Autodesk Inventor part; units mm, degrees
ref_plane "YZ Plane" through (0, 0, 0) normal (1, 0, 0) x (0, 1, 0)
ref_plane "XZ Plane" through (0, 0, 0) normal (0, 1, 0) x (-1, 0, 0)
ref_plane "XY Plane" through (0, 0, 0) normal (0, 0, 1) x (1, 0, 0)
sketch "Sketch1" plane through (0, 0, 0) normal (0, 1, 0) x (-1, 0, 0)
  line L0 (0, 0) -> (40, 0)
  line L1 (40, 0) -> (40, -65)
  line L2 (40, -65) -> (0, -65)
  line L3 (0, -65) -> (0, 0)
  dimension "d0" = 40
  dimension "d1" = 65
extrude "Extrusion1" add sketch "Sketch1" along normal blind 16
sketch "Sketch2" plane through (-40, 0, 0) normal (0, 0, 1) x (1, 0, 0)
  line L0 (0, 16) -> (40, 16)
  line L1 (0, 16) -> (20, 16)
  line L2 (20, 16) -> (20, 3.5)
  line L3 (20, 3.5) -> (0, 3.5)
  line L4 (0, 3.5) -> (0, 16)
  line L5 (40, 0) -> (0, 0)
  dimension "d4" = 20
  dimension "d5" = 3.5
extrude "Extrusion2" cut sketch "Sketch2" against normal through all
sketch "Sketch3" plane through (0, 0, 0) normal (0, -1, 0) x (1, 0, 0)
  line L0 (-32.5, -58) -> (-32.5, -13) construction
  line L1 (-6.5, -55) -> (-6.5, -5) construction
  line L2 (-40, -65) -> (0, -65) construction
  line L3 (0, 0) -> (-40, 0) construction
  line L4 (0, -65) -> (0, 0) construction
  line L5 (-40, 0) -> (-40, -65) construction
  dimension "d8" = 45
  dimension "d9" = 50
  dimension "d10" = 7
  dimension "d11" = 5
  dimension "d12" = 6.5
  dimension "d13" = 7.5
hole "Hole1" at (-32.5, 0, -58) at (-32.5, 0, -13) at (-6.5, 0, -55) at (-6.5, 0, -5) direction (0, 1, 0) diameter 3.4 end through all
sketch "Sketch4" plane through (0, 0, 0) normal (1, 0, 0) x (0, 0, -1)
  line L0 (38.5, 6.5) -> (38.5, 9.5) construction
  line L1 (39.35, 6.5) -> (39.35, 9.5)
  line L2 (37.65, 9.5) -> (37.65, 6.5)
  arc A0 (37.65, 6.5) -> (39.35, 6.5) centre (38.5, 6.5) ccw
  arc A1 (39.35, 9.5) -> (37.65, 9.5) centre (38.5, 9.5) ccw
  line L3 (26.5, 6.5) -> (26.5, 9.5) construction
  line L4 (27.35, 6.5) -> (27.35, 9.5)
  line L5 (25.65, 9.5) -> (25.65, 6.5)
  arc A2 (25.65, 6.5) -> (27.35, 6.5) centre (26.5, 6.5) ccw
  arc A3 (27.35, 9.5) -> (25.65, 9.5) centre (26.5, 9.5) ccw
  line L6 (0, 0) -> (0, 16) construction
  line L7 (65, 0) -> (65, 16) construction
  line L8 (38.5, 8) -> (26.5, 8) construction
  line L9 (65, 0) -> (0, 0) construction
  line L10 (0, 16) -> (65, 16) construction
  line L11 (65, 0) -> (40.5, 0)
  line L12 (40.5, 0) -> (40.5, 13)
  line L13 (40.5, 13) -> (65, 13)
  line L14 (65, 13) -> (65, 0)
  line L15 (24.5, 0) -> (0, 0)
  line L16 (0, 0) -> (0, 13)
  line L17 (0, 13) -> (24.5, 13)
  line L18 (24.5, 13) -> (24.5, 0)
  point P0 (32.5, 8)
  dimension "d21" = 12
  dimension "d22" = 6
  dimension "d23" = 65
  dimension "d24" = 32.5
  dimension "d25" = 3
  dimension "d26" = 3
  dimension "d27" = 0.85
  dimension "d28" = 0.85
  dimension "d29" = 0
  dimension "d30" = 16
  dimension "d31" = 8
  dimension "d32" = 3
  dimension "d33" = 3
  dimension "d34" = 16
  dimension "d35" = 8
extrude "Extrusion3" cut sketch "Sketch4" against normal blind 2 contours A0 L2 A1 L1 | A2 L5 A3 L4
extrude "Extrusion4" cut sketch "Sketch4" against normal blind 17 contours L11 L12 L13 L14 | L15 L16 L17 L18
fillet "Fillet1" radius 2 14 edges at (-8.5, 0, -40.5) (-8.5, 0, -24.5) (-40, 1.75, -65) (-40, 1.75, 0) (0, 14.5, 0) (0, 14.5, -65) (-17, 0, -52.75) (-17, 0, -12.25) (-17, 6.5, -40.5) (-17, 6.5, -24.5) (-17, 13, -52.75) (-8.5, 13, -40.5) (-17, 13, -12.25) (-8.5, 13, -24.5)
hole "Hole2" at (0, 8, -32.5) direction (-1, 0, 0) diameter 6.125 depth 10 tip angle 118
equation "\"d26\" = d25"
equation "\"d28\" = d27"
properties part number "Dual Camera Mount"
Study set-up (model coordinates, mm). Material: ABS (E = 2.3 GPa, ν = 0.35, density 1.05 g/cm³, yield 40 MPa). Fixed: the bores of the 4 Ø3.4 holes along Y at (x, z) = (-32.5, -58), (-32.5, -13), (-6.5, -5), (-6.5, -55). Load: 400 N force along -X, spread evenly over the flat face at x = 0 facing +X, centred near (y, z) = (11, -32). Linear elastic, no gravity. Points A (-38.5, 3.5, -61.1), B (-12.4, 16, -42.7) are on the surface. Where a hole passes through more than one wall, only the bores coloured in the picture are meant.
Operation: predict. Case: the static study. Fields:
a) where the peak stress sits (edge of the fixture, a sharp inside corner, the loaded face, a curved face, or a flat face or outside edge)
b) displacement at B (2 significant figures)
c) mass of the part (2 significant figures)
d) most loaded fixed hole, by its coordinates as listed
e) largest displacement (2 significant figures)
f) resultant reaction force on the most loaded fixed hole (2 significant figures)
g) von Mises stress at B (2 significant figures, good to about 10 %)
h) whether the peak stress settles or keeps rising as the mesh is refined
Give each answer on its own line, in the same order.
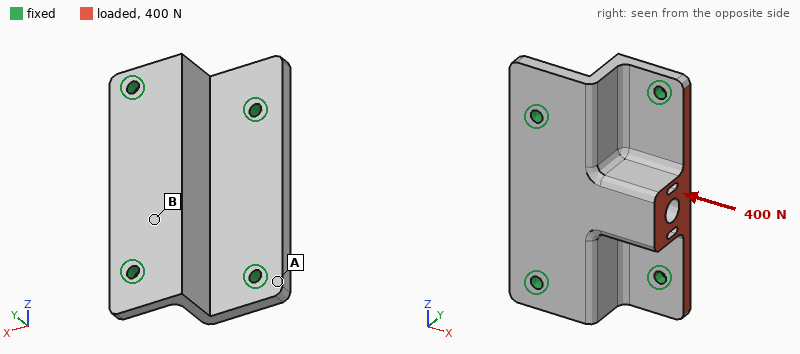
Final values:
edge of the fixture
55 µm
15 g
(-6.5, -55)
86 µm
150 N
3.7 MPa
keeps rising
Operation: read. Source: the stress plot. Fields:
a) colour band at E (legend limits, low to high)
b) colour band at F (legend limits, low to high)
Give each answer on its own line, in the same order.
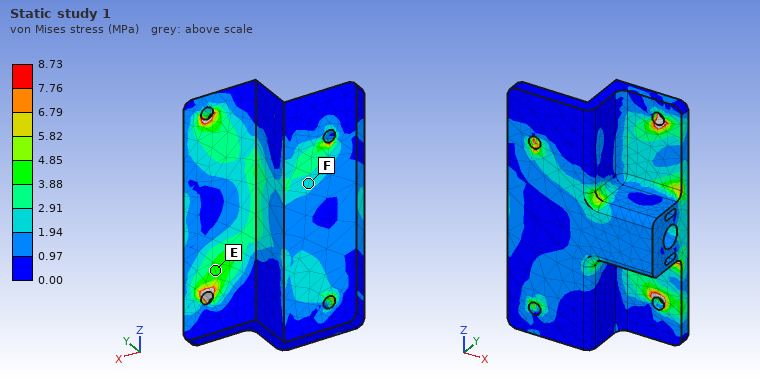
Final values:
3.88 to 4.85 MPa
1.94 to 2.91 MPa
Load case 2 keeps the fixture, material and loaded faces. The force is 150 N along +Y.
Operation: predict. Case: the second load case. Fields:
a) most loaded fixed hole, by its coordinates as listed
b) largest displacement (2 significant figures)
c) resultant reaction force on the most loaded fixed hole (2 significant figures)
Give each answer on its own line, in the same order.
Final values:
(-6.5, -55)
0.21 mm
93 N
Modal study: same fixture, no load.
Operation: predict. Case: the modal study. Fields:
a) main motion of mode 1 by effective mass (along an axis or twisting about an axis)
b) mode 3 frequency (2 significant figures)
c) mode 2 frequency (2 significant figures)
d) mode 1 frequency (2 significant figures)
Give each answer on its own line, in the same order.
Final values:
along Y
4000 Hz
3300 Hz
1900 Hz
